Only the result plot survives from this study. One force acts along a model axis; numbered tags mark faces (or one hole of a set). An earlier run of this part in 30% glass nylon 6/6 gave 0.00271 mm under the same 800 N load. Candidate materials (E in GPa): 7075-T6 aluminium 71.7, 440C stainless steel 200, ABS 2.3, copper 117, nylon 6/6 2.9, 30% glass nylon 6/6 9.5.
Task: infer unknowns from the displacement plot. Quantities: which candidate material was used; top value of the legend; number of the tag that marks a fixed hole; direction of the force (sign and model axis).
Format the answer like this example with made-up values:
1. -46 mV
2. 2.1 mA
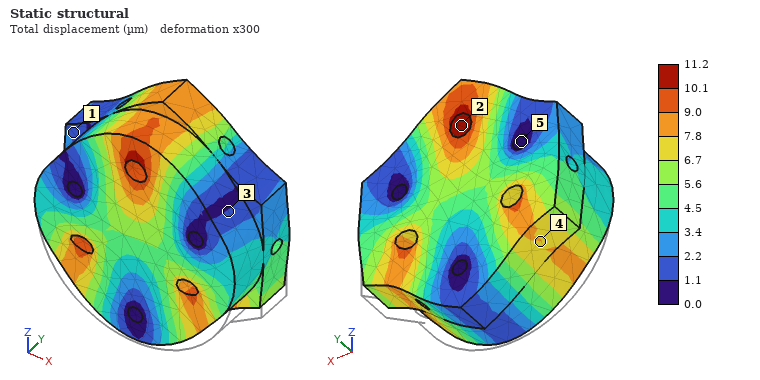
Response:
1. ABS
2. 11.2 µm
3. 5
4. +Z
